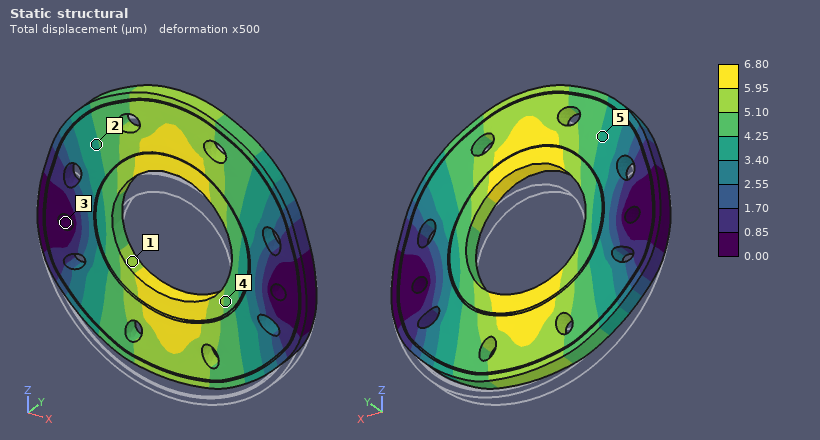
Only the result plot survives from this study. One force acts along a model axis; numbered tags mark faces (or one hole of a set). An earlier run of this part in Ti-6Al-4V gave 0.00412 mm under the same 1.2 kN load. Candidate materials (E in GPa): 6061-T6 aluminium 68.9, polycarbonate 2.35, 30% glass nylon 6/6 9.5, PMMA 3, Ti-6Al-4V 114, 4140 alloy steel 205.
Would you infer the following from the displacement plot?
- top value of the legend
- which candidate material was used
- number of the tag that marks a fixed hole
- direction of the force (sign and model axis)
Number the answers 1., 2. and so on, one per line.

1. 6.80 µm
2. 6061-T6 aluminium
3. 3
4. +Z
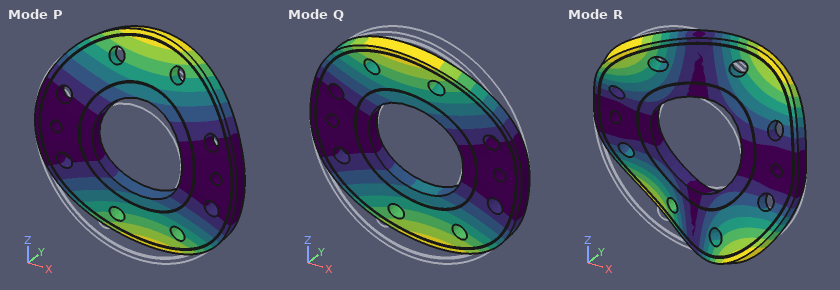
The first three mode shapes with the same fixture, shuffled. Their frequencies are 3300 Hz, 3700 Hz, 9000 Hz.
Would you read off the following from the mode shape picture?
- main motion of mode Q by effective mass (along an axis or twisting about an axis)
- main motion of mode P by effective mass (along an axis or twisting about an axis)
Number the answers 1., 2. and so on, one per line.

1. twisting about X
2. along Y
